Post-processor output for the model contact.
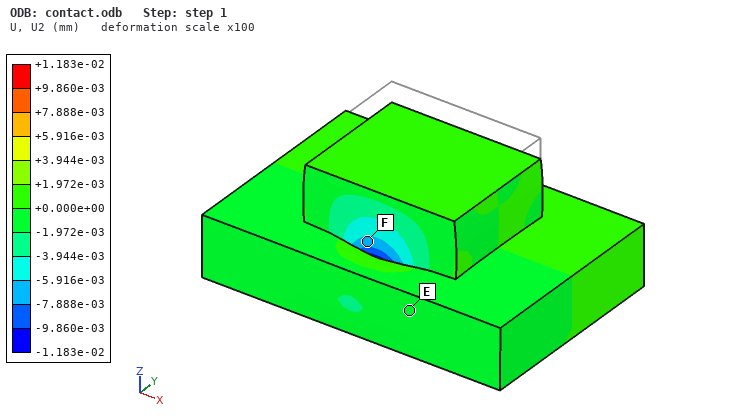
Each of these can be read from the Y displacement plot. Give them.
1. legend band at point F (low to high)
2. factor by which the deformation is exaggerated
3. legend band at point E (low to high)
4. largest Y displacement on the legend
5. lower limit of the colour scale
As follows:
-7.888e-03 to -5.916e-03 mm
100
-1.972e-03 to +0.000e+00 mm
+1.183e-02 mm
-1.183e-02 mm
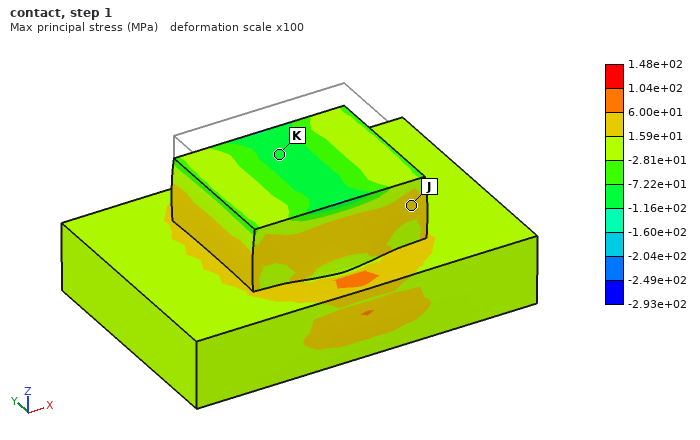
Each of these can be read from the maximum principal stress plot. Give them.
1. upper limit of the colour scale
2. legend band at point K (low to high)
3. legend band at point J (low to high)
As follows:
1.48e+02 MPa
-1.16e+02 to -7.22e+01 MPa
1.59e+01 to 6.00e+01 MPa
